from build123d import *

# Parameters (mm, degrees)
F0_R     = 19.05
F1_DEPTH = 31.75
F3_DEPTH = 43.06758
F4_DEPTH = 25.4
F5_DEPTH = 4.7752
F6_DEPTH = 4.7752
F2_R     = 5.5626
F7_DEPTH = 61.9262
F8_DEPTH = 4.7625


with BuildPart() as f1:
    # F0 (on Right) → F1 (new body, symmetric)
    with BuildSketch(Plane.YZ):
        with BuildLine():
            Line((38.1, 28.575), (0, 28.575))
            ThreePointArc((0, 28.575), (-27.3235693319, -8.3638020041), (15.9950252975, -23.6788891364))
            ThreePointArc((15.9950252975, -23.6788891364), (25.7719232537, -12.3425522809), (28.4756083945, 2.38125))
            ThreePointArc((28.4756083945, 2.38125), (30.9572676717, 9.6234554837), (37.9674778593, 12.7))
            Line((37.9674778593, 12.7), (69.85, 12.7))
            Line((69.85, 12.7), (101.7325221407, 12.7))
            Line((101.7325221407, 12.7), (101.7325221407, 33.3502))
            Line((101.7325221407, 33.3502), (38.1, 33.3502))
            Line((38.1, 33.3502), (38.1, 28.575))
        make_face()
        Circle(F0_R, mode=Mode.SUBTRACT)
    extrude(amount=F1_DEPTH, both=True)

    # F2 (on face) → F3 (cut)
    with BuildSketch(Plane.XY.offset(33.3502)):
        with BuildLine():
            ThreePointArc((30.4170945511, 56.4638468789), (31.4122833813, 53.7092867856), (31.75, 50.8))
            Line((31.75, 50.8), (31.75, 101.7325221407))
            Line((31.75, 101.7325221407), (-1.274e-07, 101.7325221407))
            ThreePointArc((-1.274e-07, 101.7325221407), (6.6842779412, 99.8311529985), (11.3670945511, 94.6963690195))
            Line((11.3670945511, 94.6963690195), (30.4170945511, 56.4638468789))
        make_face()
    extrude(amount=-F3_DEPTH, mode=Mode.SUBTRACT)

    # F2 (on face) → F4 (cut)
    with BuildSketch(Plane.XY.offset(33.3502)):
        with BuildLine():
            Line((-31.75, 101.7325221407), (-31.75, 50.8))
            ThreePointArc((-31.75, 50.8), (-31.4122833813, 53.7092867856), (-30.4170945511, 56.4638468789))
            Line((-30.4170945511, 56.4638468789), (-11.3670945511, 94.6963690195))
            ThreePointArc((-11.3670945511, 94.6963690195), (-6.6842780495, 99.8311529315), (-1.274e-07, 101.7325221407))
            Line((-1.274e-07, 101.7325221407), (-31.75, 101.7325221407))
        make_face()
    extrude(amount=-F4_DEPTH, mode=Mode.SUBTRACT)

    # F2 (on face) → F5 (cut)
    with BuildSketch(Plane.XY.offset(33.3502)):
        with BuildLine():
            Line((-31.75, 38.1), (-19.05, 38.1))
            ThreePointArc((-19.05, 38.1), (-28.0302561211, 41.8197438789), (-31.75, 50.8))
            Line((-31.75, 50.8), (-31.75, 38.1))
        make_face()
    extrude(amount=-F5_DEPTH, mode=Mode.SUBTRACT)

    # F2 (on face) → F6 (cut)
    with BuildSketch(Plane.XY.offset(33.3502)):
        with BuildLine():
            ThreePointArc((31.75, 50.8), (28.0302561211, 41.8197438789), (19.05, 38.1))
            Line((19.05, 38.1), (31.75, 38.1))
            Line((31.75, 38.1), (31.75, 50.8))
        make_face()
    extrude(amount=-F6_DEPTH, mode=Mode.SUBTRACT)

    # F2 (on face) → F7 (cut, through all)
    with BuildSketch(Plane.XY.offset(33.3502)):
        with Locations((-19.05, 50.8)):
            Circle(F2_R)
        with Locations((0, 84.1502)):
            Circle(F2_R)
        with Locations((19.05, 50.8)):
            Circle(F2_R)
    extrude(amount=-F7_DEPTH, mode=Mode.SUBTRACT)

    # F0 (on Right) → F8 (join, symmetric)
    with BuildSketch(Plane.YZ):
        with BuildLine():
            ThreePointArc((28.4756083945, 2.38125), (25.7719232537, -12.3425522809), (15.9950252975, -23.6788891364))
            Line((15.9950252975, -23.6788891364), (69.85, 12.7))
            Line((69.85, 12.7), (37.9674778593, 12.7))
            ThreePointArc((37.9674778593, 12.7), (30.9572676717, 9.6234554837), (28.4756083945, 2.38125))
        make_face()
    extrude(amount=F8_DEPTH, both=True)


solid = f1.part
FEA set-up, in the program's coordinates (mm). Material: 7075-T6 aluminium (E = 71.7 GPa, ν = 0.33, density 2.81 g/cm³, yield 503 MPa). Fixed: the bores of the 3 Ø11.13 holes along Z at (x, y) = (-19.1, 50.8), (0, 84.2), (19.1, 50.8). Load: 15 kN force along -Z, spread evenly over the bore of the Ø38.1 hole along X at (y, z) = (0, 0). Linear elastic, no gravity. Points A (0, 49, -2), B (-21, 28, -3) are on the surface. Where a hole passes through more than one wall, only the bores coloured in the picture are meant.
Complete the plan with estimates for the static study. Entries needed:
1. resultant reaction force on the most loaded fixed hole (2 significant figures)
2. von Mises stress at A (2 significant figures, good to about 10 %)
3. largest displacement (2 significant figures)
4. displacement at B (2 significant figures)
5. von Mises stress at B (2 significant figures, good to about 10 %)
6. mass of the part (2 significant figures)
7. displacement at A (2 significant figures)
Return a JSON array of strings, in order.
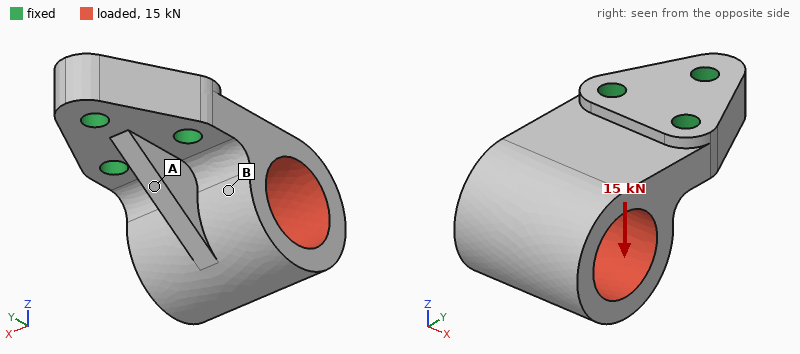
["10 kN", "120 MPa", "0.40 mm", "0.11 mm", "17 MPa", "480 g", "0.066 mm"]
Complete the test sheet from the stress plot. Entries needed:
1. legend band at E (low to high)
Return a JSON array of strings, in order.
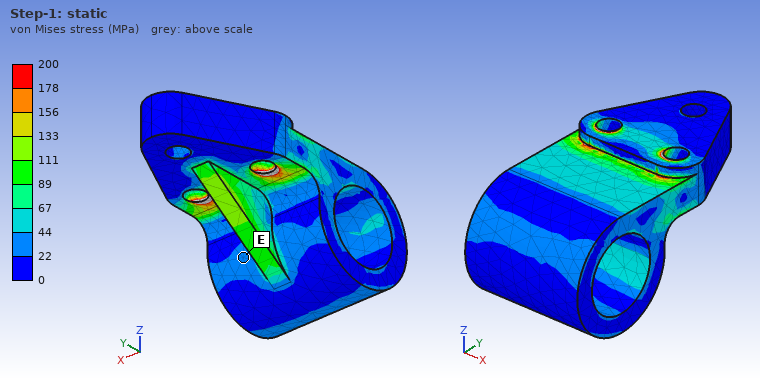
["22 to 44 MPa"]
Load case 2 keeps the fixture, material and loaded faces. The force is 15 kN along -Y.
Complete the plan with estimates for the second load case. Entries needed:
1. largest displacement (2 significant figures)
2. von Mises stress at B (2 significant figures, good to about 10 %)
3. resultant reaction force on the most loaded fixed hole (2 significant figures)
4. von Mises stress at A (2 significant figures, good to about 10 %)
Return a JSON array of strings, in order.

["0.20 mm", "21 MPa", "6.1 kN", "83 MPa"]
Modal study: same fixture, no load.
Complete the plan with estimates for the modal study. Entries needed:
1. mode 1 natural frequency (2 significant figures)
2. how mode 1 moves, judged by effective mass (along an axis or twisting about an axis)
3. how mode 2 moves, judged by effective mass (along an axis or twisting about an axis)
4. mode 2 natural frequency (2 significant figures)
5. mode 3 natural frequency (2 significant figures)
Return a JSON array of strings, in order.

["2000 Hz", "along Z", "along X", "3700 Hz", "6000 Hz"]
